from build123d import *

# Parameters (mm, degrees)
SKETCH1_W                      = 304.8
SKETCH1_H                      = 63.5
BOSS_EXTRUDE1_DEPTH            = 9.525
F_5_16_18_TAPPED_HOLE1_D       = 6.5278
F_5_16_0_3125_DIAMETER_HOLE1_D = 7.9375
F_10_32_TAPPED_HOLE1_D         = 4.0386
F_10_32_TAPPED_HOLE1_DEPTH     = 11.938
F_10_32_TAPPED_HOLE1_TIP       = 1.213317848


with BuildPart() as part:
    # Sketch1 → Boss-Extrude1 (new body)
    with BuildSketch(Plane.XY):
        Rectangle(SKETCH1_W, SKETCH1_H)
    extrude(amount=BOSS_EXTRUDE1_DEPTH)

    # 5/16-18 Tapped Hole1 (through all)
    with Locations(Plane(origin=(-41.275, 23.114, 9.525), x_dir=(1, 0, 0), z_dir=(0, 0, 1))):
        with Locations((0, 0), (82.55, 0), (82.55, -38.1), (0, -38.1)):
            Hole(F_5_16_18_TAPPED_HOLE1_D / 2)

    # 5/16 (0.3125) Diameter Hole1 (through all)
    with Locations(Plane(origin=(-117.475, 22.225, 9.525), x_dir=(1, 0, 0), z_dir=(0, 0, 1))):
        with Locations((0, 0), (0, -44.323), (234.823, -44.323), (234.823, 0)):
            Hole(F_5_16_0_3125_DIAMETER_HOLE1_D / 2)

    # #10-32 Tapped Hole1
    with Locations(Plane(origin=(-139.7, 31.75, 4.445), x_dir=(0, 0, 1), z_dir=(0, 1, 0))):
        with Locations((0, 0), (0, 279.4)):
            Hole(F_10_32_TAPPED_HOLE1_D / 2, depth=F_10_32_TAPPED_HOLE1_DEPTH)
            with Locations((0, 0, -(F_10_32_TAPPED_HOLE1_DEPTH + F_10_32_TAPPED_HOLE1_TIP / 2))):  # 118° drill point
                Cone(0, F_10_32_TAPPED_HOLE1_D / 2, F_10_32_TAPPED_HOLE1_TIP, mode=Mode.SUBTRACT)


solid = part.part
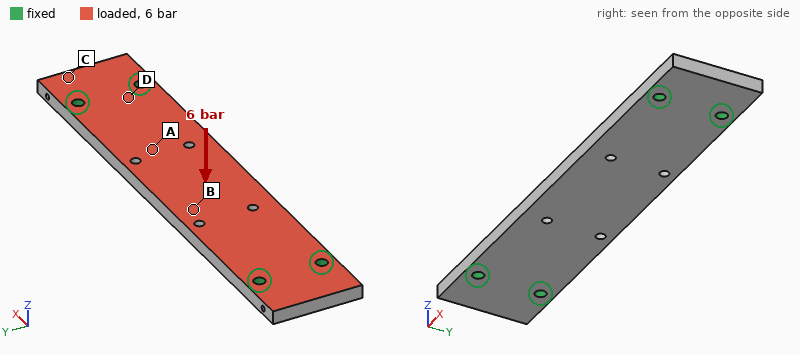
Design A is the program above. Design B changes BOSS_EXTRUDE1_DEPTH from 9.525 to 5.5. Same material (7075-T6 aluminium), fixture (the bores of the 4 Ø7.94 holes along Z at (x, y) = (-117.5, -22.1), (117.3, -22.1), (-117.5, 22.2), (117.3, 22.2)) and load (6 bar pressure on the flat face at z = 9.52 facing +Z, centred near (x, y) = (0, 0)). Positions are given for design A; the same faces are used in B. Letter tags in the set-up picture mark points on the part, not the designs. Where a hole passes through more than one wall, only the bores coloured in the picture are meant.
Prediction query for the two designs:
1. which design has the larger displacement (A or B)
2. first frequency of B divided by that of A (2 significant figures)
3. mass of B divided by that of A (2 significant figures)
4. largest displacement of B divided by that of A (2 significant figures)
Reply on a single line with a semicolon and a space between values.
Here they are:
B; 0.59; 0.58; 4.9
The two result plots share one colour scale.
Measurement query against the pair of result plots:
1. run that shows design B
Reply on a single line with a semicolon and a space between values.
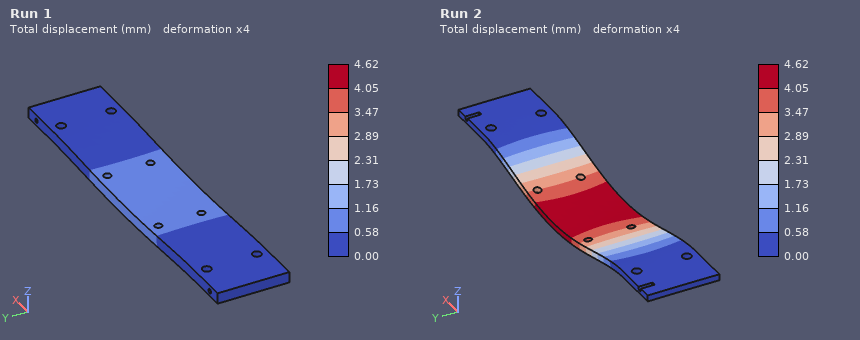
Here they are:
Run 2
